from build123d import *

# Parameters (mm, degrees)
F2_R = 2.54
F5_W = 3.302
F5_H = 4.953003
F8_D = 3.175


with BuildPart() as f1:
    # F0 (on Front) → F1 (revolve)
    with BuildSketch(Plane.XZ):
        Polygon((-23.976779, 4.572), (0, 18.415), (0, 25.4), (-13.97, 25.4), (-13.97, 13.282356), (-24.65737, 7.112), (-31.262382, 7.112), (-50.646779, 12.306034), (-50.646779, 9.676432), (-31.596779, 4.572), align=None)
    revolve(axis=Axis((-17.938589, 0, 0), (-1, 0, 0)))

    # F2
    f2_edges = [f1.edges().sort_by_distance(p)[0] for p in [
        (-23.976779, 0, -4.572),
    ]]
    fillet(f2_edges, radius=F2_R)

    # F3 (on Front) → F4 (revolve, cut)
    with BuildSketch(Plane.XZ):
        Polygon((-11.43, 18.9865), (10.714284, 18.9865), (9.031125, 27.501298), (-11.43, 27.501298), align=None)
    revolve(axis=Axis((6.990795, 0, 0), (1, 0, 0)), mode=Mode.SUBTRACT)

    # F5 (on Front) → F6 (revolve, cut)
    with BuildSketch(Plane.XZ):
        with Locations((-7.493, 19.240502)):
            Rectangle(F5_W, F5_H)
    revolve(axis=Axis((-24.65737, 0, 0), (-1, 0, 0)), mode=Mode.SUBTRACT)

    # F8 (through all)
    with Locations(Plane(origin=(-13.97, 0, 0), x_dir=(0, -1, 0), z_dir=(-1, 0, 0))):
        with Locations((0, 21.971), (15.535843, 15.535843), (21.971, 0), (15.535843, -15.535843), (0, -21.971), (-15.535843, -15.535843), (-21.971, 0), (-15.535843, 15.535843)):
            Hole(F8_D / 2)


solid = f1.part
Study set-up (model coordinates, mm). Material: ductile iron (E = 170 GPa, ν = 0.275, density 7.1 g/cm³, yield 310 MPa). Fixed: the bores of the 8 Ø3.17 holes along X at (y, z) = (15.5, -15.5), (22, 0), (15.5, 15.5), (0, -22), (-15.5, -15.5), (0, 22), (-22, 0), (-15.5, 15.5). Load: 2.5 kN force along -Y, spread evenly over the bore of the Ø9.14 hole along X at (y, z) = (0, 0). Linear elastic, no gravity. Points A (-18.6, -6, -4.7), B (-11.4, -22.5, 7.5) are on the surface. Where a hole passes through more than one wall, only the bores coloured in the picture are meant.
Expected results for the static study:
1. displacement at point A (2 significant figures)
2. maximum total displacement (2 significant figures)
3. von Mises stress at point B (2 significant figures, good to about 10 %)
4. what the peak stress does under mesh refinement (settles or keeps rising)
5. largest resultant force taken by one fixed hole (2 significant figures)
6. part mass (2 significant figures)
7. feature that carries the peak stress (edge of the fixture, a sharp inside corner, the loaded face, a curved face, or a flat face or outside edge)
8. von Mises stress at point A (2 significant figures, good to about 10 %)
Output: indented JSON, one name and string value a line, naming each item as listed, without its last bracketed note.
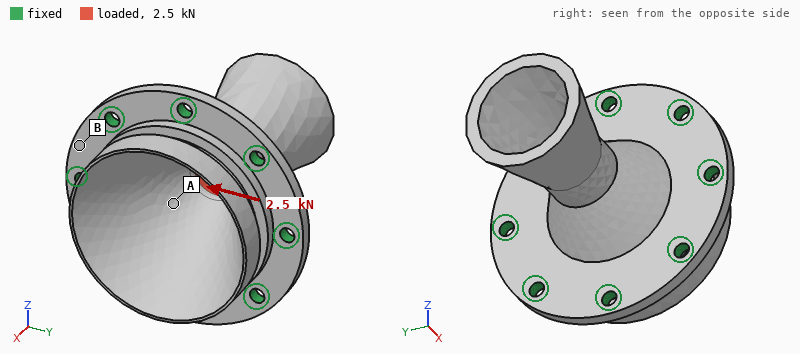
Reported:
{
  "displacement at point A": "5.3 µm",
  "maximum total displacement": "31 µm",
  "von Mises stress at point B": "14 MPa",
  "what the peak stress does under mesh refinement": "keeps rising",
  "largest resultant force taken by one fixed hole": "600 N",
  "part mass": "91 g",
  "feature that carries the peak stress": "edge of the fixture",
  "von Mises stress at point A": "30 MPa"
}
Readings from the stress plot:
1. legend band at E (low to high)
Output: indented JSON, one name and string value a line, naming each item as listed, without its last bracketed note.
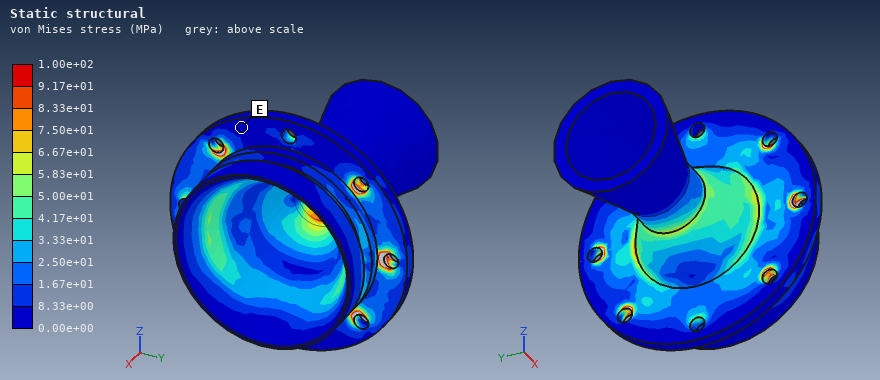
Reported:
{
  "legend band at E": "0.00e+00 to 8.33e+00 MPa"
}
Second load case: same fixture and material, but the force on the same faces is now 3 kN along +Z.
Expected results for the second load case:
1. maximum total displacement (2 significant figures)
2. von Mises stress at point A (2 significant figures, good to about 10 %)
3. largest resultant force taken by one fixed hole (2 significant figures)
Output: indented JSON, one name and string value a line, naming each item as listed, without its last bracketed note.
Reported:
{
  "maximum total displacement": "37 µm",
  "von Mises stress at point A": "36 MPa",
  "largest resultant force taken by one fixed hole": "720 N"
}
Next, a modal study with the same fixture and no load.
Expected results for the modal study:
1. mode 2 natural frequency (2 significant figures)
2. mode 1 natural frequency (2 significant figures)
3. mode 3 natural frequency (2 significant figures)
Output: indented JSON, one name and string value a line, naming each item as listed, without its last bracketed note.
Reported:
{
  "mode 2 natural frequency": "6000 Hz",
  "mode 1 natural frequency": "6000 Hz",
  "mode 3 natural frequency": "14 kHz"
}
